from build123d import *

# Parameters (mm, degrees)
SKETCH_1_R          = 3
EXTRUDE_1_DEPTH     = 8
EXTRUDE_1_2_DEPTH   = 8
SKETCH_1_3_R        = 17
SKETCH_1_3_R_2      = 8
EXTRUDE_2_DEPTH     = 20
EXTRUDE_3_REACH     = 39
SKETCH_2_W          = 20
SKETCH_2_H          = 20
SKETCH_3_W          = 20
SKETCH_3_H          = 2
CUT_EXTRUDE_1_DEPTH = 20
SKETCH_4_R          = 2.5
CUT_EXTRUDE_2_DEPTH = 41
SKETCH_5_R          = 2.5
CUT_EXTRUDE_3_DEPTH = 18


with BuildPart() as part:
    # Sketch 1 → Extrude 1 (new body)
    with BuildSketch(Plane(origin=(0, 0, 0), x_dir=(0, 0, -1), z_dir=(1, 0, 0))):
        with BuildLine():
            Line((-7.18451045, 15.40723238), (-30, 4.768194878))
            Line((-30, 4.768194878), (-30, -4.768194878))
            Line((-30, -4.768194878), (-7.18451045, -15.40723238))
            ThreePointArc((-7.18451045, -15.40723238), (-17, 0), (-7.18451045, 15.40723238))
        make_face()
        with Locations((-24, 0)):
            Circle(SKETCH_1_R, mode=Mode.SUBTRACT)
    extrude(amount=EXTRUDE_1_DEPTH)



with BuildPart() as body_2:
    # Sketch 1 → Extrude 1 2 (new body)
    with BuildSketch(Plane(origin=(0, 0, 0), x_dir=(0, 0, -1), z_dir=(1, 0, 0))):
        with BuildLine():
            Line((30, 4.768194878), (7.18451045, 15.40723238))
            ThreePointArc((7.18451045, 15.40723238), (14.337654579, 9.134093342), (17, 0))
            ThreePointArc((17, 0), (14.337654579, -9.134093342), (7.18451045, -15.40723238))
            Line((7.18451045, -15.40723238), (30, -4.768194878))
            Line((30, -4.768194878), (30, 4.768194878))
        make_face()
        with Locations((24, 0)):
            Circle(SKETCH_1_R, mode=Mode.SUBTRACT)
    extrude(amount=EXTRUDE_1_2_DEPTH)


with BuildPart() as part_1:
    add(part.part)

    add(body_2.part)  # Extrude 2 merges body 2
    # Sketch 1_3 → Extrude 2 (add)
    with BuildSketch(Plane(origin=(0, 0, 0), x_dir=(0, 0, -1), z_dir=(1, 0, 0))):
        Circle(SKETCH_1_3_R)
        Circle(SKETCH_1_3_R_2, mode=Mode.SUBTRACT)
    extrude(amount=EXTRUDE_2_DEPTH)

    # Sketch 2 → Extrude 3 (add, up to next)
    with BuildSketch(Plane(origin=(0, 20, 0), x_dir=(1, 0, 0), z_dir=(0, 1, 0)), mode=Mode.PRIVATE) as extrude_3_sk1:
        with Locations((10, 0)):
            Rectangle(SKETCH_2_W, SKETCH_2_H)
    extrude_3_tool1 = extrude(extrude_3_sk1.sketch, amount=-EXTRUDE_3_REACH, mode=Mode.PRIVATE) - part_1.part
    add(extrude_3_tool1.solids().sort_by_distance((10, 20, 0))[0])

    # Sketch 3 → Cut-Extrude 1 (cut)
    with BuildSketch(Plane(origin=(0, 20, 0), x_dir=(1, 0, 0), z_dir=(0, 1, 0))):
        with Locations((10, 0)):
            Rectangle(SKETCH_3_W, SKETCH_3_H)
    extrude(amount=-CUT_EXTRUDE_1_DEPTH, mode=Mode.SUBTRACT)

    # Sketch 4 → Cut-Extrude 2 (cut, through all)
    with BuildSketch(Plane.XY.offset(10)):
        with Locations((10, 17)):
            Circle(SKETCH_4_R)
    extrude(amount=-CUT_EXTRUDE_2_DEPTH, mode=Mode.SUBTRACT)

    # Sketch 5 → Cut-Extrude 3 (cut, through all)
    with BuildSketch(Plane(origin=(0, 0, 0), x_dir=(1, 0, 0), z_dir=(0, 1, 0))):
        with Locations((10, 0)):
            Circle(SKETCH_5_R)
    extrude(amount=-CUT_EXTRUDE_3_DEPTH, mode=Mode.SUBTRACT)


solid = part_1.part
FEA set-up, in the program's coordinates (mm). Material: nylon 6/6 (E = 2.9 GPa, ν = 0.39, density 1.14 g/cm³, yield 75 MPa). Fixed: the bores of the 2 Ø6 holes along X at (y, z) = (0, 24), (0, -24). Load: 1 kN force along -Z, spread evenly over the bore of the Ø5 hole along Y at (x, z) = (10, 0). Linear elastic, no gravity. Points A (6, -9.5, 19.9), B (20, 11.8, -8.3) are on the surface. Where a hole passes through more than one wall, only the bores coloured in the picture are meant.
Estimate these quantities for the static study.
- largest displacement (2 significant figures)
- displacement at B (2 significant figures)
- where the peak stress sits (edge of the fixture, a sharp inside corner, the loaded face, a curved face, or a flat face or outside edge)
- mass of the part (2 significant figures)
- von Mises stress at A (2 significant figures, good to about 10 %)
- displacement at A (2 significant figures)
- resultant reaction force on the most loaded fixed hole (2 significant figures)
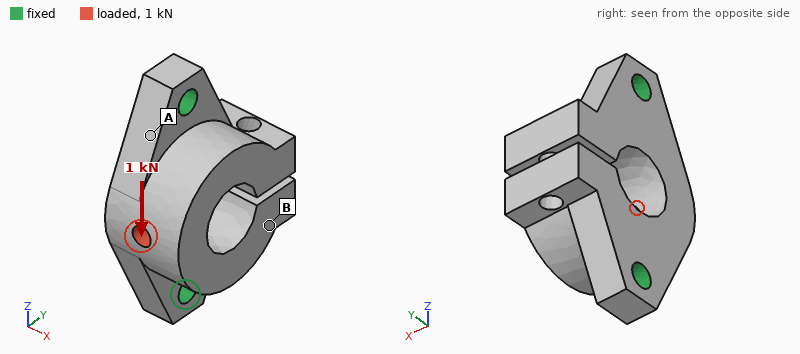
74 µm
20 µm
the loaded face
21 g
5.4 MPa
22 µm
570 N
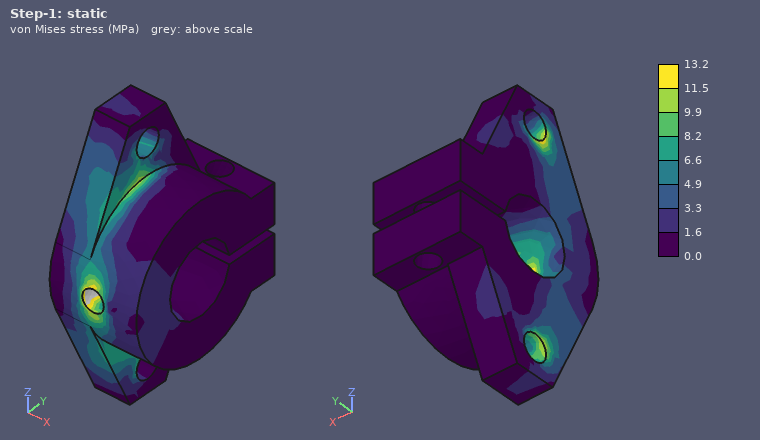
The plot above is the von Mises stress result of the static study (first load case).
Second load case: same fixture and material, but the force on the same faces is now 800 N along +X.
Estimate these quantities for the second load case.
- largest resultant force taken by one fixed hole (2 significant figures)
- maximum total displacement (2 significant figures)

420 N
0.50 mm
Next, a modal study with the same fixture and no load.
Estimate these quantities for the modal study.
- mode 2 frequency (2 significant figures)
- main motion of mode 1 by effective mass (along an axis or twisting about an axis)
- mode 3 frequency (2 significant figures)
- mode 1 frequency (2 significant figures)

2600 Hz
along Y
2800 Hz
2200 Hz
